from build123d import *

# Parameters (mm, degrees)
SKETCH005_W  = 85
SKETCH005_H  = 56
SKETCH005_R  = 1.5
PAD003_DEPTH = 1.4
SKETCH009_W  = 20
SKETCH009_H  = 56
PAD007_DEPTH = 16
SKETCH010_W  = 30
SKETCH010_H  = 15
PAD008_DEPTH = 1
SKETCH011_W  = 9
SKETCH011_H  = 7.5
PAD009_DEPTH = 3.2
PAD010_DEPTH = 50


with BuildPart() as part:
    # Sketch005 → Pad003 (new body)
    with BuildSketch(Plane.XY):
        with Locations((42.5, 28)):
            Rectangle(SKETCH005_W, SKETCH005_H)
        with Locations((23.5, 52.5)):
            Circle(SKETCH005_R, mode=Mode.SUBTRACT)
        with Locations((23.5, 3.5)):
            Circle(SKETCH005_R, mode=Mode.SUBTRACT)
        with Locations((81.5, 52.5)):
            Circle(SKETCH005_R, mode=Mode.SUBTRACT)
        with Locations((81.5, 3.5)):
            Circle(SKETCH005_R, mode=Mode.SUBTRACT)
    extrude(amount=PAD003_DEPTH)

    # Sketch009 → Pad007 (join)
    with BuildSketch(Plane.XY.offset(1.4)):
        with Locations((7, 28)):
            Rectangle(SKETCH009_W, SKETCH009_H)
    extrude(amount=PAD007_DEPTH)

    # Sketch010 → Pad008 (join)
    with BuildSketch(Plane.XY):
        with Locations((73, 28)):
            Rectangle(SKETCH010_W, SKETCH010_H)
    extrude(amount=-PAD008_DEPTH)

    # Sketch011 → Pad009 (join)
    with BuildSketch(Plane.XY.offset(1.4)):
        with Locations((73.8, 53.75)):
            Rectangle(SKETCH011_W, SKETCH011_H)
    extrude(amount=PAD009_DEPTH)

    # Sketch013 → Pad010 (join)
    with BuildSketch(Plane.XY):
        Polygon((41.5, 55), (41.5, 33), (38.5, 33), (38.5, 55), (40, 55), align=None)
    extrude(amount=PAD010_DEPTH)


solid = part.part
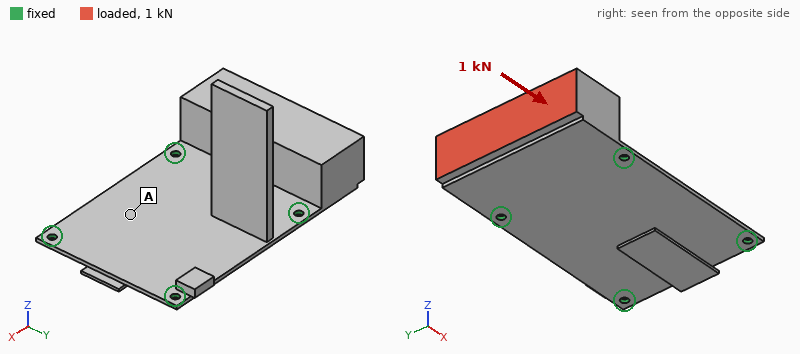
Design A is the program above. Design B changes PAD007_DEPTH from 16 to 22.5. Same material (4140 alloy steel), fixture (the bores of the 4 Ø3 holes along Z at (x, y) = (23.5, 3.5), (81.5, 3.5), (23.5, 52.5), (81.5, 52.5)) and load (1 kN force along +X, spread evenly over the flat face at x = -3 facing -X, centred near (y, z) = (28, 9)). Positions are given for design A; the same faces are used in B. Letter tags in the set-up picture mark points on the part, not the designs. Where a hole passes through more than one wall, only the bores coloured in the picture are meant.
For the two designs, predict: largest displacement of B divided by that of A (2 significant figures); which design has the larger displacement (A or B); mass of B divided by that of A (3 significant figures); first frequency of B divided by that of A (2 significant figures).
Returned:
1.6
B
1.26
0.76
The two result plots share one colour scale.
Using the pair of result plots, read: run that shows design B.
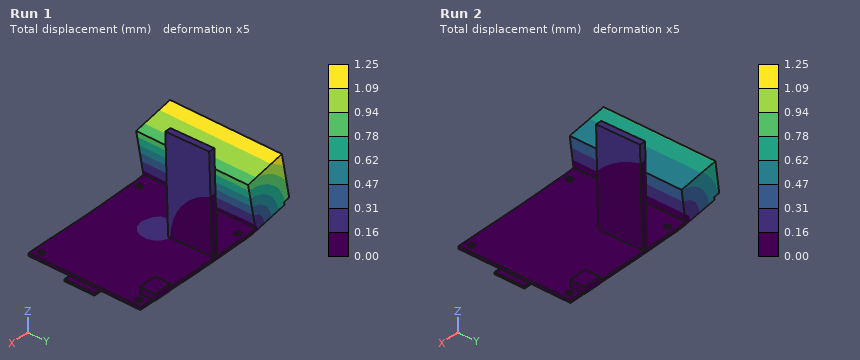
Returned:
Run 1
